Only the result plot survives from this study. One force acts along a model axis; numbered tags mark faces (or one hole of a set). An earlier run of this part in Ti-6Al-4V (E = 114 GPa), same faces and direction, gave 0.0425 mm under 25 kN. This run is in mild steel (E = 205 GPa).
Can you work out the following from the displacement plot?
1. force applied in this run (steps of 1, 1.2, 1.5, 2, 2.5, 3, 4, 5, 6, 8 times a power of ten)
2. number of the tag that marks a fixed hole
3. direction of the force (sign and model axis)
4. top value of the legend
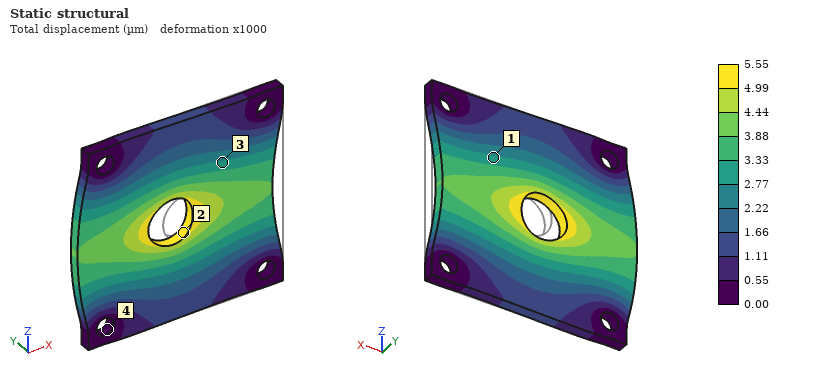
6 kN
4
-X
5.55 µm
